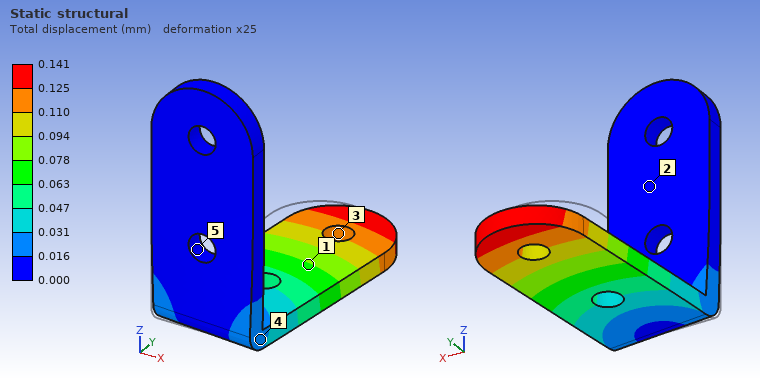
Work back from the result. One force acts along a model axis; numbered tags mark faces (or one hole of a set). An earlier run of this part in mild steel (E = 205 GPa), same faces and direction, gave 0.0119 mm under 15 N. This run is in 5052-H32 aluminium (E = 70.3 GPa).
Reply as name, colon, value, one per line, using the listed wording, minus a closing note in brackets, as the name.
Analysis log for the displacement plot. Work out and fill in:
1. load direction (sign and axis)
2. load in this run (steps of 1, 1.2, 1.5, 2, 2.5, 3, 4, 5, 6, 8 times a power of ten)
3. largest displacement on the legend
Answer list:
load direction: +X
load in this run: 60 N
largest displacement on the legend: 0.141 mm
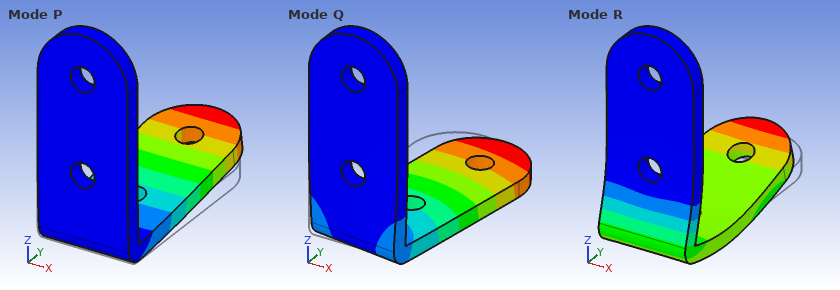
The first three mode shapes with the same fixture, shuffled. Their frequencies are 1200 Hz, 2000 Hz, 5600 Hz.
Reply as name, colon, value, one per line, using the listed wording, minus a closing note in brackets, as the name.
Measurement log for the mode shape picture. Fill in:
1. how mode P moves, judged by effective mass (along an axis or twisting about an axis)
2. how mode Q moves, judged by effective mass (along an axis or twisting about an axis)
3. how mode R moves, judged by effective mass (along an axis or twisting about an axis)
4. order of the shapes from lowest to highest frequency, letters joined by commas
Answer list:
how mode P moves, judged by effective mass: along Z
how mode Q moves, judged by effective mass: along X
how mode R moves, judged by effective mass: along Y
order of the shapes from lowest to highest frequency, letters joined by commas: P, Q, R
